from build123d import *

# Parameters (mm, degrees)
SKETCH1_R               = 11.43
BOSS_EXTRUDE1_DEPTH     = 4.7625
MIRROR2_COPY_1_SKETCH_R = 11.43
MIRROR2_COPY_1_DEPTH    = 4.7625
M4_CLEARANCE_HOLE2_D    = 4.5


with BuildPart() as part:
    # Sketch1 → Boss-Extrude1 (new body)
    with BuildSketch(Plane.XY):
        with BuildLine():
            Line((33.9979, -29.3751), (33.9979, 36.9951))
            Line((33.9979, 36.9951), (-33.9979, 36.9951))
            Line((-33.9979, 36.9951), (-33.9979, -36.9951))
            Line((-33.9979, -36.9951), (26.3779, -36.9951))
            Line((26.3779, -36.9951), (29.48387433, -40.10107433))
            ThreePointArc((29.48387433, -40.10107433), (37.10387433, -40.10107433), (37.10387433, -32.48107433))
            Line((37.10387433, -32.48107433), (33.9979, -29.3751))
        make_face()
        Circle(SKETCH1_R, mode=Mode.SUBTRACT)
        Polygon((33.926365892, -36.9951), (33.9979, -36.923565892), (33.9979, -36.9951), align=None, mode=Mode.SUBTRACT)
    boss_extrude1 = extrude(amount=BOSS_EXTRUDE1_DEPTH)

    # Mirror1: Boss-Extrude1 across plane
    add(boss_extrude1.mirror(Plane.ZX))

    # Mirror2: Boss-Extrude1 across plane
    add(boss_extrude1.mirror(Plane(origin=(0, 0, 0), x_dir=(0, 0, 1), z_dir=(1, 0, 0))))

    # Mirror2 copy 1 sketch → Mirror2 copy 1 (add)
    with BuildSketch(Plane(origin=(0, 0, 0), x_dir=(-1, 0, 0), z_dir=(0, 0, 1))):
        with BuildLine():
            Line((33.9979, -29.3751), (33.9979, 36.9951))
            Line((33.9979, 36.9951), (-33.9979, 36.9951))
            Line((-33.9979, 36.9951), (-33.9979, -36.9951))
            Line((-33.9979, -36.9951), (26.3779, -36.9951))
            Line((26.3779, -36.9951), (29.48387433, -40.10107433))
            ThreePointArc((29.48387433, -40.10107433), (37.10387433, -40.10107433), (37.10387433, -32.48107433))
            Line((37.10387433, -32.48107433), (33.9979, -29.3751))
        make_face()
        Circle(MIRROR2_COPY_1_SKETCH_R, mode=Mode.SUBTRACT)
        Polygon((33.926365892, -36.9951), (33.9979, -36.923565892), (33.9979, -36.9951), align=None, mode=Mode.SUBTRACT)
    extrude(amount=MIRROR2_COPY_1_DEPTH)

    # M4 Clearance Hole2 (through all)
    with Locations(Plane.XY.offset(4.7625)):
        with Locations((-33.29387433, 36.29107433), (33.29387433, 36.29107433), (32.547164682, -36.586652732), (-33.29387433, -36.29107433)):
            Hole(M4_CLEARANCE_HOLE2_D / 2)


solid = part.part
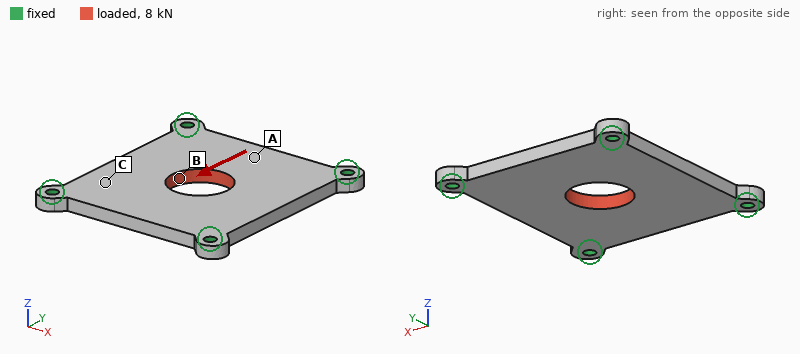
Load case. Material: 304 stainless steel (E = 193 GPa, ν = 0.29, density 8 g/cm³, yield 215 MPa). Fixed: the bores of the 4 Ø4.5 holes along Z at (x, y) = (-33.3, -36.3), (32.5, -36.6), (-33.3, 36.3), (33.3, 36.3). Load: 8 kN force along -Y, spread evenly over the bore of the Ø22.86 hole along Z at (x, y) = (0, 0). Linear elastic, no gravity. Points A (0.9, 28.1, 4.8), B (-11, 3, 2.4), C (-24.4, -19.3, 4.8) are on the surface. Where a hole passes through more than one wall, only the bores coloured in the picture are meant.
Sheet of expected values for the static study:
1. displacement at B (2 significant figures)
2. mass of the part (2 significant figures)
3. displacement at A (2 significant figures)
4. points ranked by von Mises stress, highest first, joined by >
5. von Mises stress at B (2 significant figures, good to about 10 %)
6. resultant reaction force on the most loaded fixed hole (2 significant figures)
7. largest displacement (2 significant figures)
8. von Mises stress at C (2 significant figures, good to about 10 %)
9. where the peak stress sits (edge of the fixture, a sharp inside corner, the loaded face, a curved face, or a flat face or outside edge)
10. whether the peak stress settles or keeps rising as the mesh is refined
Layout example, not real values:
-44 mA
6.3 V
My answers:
6.8 µm
180 g
6.7 µm
B > C > A
41 MPa
2.4 kN
7.8 µm
24 MPa
edge of the fixture
keeps rising
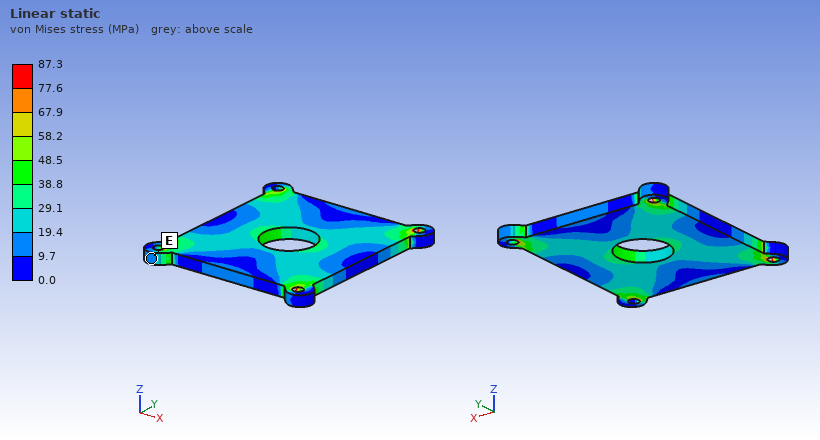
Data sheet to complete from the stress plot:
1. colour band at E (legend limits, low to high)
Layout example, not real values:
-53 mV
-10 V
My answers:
9.7 to 19.4 MPa
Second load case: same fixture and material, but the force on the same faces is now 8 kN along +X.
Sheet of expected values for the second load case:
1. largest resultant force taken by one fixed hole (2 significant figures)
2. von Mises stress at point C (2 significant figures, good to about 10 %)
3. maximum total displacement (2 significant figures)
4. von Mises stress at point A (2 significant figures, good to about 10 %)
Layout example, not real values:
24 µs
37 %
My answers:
2.4 kN
22 MPa
8.9 µm
17 MPa
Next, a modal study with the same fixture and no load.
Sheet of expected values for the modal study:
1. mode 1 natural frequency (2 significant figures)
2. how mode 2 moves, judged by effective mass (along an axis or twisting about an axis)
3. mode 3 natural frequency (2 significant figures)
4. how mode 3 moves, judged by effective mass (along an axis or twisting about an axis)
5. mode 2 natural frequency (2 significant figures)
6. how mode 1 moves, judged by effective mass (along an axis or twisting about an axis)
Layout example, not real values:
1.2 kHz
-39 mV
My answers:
2900 Hz
twisting about Y
5500 Hz
twisting about X
5100 Hz
along Z
